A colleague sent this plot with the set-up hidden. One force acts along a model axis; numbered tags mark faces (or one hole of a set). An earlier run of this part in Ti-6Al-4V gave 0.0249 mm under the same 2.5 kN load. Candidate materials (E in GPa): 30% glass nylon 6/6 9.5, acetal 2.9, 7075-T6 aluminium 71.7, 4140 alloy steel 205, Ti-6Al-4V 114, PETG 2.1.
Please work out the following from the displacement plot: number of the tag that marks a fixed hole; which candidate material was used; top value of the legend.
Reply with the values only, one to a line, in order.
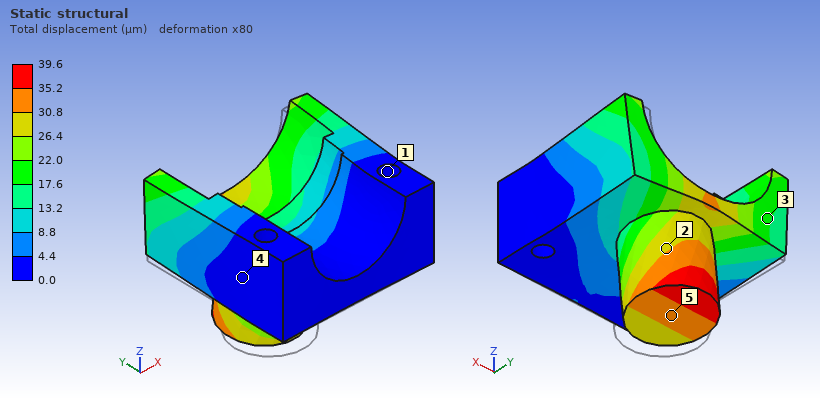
1
7075-T6 aluminium
39.6 µm
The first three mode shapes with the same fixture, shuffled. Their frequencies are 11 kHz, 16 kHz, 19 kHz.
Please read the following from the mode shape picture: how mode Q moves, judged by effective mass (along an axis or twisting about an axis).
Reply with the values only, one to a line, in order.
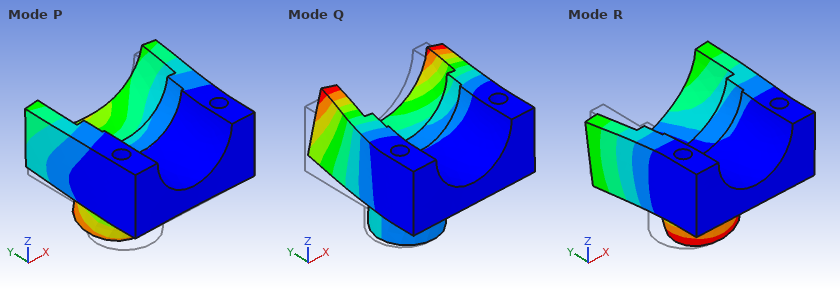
along X
